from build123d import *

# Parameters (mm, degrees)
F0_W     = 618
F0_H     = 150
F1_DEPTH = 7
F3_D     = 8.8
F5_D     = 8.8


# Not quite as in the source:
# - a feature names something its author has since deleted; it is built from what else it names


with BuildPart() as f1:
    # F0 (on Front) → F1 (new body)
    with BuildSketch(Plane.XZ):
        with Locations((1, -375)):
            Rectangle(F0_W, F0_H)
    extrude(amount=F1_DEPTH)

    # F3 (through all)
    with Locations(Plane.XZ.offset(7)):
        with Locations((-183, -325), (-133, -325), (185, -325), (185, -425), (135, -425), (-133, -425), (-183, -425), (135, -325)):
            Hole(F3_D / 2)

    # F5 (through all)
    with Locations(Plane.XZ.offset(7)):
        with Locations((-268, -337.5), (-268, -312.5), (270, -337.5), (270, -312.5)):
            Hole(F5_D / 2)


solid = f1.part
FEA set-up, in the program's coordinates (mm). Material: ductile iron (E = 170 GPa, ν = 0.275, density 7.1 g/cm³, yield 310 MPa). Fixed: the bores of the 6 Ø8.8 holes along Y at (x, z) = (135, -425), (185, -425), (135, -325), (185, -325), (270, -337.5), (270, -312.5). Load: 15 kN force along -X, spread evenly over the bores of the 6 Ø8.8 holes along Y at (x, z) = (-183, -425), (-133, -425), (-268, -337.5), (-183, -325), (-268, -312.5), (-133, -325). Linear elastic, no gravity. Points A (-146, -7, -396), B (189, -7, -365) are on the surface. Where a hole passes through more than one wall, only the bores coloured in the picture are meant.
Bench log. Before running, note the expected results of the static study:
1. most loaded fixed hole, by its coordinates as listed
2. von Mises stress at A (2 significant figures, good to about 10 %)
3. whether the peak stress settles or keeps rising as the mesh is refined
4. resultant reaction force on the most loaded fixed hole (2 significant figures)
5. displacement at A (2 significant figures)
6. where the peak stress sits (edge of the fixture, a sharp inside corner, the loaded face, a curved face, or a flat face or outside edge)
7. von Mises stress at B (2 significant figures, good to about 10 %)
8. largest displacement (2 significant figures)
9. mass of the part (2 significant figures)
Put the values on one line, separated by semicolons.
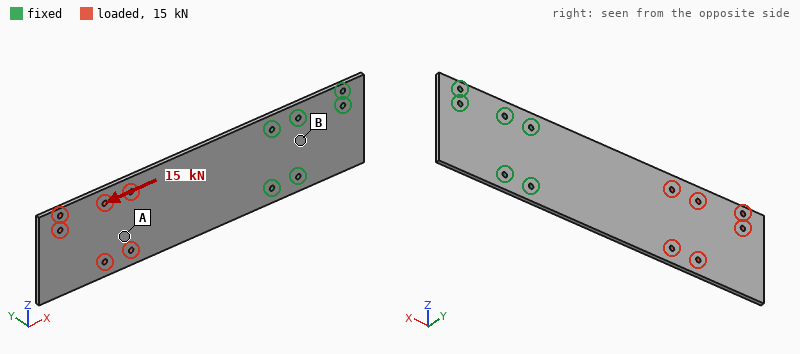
(135, -325); 8.6 MPa; keeps rising; 7.3 kN; 37 µm; edge of the fixture; 3.6 MPa; 94 µm; 4.6 kg
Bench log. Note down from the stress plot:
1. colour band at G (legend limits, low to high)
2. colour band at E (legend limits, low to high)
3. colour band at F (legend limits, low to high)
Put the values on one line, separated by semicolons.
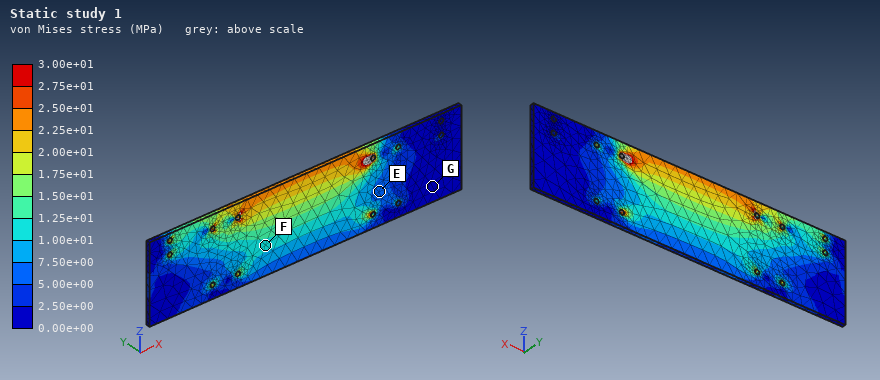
0.00e+00 to 2.50e+00 MPa; 5.00e+00 to 7.50e+00 MPa; 1.00e+01 to 1.25e+01 MPa
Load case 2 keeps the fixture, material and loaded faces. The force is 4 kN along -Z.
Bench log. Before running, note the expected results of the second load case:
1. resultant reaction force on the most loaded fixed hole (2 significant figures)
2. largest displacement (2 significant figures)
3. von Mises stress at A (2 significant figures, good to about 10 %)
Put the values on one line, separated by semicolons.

10 kN; 0.27 mm; 7.7 MPa
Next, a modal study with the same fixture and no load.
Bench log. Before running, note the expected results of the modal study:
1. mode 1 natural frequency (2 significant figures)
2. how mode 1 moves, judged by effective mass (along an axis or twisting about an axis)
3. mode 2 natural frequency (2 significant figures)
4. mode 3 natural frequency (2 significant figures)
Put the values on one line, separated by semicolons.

28 Hz; along Y; 170 Hz; 180 Hz
